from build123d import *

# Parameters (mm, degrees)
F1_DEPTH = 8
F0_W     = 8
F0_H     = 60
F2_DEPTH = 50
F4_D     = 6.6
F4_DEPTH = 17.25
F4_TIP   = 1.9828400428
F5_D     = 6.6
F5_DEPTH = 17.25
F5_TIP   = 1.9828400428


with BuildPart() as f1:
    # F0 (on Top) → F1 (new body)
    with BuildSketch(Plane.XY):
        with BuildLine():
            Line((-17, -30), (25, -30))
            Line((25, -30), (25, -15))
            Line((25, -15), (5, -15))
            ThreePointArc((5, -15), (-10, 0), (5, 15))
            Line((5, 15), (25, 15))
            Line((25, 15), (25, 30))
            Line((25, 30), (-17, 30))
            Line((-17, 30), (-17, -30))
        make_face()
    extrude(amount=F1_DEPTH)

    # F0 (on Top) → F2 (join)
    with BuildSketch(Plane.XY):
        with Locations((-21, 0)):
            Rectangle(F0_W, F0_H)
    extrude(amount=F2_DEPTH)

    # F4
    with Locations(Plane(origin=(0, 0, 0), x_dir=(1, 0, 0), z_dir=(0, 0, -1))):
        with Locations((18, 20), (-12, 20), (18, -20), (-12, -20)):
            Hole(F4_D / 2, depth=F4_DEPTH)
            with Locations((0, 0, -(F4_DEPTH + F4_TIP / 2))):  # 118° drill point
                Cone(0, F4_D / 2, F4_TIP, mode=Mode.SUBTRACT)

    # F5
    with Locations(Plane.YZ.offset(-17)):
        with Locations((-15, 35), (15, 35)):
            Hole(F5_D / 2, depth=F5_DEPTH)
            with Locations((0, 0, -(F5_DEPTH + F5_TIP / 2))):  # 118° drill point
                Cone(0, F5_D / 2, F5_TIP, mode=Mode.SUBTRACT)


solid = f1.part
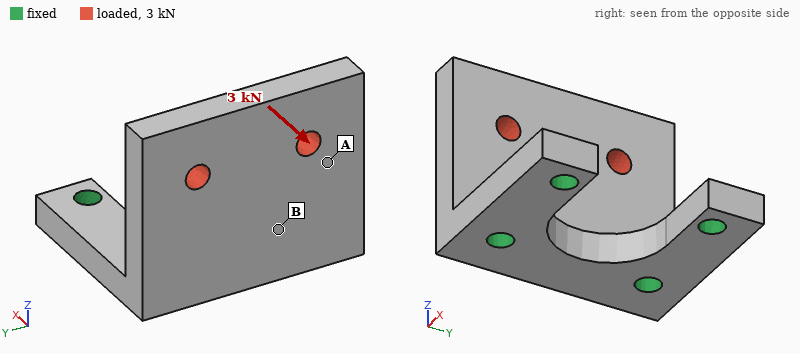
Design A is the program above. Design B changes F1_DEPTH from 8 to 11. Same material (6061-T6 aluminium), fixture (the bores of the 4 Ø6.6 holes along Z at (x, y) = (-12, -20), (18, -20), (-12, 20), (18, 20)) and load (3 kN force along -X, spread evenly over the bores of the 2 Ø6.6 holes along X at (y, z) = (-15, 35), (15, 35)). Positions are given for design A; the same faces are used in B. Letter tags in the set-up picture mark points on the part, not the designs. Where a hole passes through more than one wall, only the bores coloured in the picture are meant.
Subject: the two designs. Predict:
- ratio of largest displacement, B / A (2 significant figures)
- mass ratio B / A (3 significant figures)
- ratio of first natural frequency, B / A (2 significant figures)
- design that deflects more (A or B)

0.63
1.12
1.3
A
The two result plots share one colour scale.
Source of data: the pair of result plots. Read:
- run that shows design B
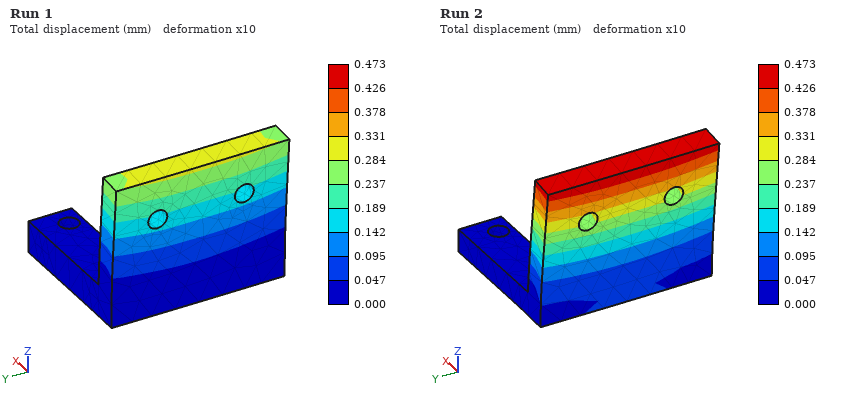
Run 1
